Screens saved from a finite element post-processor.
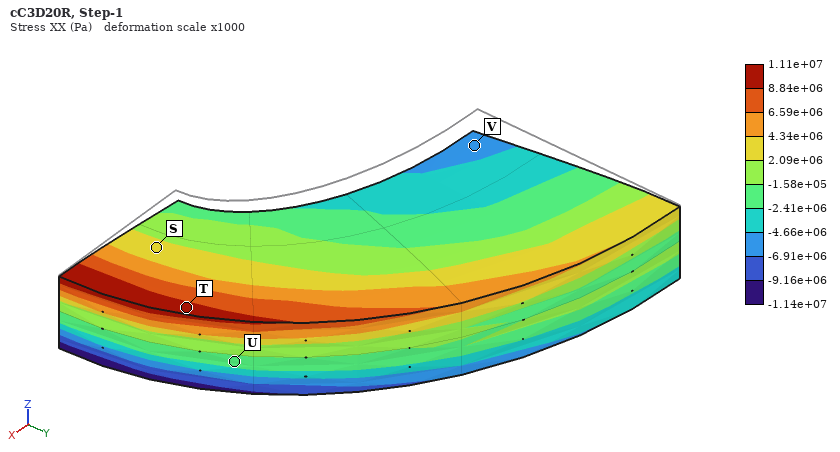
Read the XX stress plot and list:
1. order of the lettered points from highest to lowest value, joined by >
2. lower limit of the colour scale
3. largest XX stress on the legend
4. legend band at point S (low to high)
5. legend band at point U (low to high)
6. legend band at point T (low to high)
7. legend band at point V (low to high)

T > S > U > V
-1.14e+07 Pa
1.11e+07 Pa
2.09e+06 to 4.34e+06 Pa
-2.41e+06 to -1.58e+05 Pa
8.84e+06 to 1.11e+07 Pa
-6.91e+06 to -4.66e+06 Pa
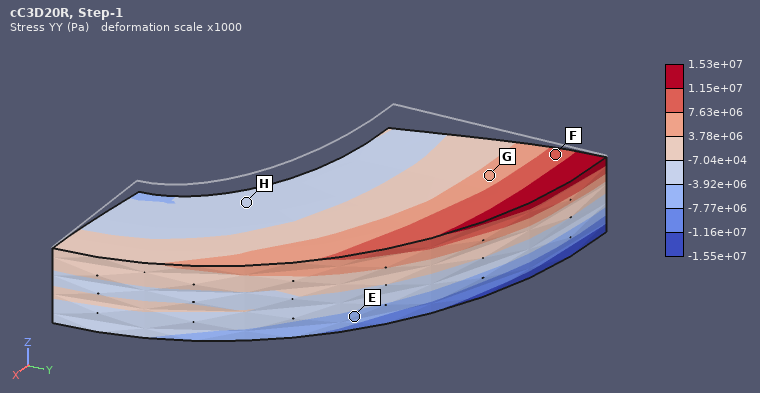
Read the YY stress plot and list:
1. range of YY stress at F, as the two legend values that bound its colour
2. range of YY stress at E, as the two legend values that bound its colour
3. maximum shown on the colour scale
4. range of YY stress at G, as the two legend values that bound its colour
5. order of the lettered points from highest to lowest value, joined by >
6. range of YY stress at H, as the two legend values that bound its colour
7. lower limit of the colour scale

7.63e+06 to 1.15e+07 Pa
-7.77e+06 to -3.92e+06 Pa
1.53e+07 Pa
3.78e+06 to 7.63e+06 Pa
F > G > H > E
-3.92e+06 to -7.04e+04 Pa
-1.55e+07 Pa
